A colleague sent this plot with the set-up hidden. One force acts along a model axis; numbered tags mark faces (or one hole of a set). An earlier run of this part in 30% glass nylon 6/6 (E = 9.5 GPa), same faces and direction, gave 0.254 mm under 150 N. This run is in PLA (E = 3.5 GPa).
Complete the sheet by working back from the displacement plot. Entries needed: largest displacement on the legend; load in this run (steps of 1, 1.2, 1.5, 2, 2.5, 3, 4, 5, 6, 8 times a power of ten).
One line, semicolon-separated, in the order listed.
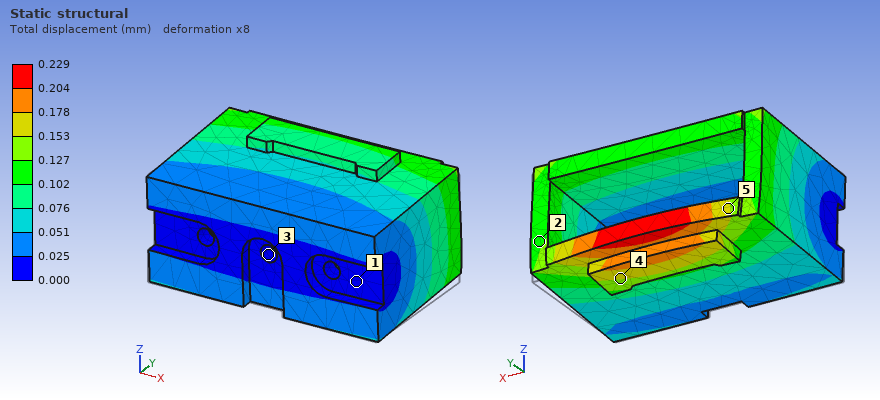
0.229 mm; 50 N
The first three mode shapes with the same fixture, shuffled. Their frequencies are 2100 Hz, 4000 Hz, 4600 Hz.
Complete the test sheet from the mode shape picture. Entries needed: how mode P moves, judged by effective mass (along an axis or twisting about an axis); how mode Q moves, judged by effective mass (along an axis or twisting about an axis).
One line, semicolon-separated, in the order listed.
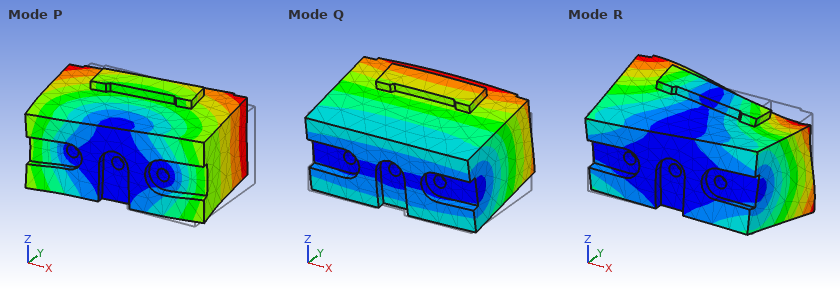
along X; along Z
